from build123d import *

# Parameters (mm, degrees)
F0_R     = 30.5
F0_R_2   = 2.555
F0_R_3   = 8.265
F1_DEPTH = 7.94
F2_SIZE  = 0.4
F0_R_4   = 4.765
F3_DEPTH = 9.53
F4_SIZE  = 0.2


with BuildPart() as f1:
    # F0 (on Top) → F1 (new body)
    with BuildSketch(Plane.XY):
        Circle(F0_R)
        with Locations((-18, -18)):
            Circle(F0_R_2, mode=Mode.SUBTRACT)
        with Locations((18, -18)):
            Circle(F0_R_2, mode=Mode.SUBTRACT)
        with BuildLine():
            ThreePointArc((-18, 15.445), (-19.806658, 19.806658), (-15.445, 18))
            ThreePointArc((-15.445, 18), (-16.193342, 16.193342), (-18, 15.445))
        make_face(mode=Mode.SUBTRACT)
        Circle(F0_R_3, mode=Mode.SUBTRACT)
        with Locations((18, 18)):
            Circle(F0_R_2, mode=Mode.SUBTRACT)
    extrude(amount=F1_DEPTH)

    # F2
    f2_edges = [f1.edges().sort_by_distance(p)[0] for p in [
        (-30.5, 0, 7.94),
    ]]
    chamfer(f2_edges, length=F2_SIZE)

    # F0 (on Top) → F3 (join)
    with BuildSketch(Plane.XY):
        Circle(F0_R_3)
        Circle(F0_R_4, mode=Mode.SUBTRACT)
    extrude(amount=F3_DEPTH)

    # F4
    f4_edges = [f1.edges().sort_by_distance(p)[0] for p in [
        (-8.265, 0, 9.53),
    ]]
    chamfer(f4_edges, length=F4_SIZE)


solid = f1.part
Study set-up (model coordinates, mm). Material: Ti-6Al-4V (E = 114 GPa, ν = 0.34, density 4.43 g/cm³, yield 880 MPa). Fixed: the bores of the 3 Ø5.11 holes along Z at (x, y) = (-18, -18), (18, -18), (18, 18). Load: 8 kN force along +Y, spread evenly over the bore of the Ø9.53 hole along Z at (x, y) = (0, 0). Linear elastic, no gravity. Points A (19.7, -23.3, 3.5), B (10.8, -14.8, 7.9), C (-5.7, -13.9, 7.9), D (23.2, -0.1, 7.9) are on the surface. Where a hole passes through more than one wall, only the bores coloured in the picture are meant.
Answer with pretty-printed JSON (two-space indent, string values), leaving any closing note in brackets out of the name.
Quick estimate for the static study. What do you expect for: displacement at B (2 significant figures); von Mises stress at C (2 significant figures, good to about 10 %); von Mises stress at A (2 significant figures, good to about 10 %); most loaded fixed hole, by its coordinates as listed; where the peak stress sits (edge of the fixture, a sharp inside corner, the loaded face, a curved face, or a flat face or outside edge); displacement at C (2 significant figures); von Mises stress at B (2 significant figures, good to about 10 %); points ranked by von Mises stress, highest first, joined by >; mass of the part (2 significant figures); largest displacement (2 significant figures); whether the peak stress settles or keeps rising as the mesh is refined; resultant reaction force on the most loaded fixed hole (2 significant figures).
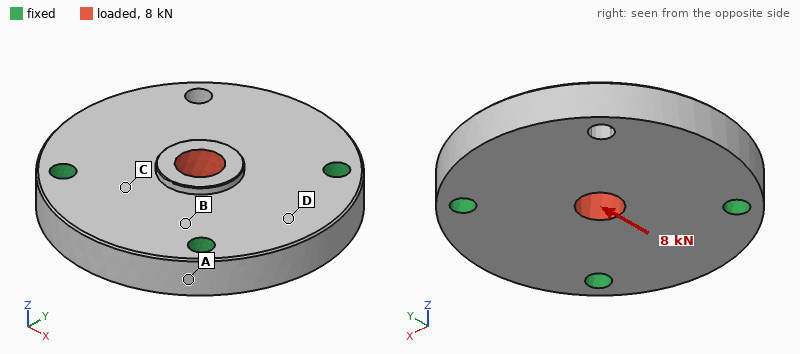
{
  "displacement at B": "2.2 µm",
  "von Mises stress at C": "19 MPa",
  "von Mises stress at A": "11 MPa",
  "most loaded fixed hole, by its coordinates as listed": "(-18, -18)",
  "where the peak stress sits": "edge of the fixture",
  "displacement at C": "4.0 µm",
  "von Mises stress at B": "26 MPa",
  "points ranked by von Mises stress, highest first, joined by >": "B > C > A > D",
  "mass of the part": "98 g",
  "largest displacement": "8.0 µm",
  "whether the peak stress settles or keeps rising as the mesh is refined": "keeps rising",
  "resultant reaction force on the most loaded fixed hole": "3.4 kN"
}
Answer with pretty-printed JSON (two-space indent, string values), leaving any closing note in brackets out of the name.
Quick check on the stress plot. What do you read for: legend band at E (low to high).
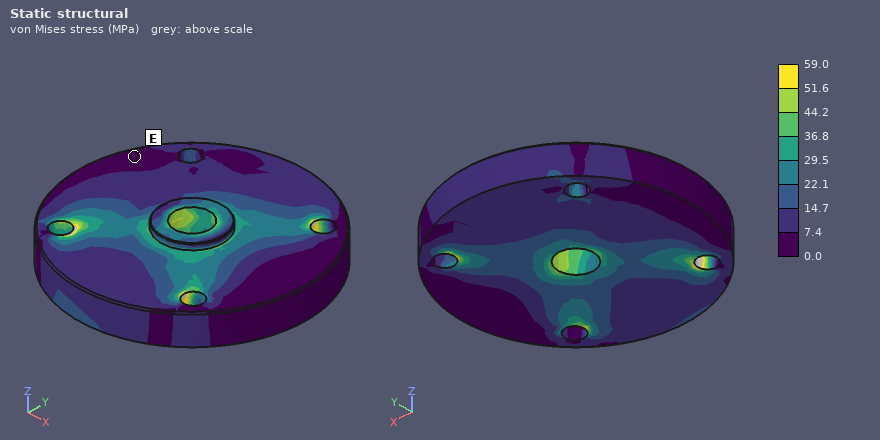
{
  "legend band at E": "0.0 to 7.4 MPa"
}
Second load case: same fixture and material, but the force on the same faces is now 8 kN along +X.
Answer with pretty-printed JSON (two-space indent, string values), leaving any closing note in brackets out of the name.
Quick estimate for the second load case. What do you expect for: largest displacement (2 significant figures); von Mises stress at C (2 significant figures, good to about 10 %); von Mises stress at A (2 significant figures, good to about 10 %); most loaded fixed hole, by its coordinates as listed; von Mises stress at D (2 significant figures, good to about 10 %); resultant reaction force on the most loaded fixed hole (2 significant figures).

{
  "largest displacement": "8.1 µm",
  "von Mises stress at C": "19 MPa",
  "von Mises stress at A": "8.4 MPa",
  "most loaded fixed hole, by its coordinates as listed": "(18, 18)",
  "von Mises stress at D": "7.9 MPa",
  "resultant reaction force on the most loaded fixed hole": "3.4 kN"
}
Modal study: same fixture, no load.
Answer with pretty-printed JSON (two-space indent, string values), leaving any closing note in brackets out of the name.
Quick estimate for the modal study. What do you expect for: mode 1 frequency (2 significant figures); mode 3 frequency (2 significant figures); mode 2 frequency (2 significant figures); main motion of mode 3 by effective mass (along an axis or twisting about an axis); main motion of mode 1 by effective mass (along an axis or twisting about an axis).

{
  "mode 1 frequency": "6600 Hz",
  "mode 3 frequency": "19 kHz",
  "mode 2 frequency": "16 kHz",
  "main motion of mode 3 by effective mass": "along Z",
  "main motion of mode 1 by effective mass": "along Z"
}
